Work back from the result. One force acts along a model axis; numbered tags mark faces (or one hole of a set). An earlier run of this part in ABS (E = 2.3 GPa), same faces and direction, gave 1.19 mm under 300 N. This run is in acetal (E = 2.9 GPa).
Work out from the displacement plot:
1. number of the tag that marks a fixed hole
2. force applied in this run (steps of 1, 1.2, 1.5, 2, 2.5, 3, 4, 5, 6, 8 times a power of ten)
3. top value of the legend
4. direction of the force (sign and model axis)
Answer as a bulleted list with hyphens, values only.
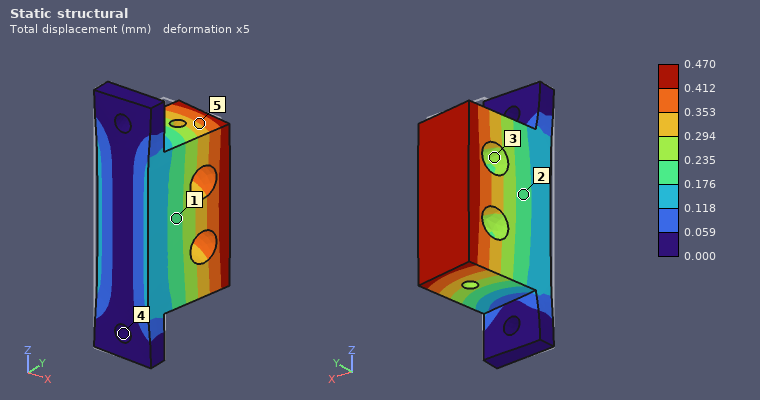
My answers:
- 4
- 150 N
- 0.470 mm
- +X
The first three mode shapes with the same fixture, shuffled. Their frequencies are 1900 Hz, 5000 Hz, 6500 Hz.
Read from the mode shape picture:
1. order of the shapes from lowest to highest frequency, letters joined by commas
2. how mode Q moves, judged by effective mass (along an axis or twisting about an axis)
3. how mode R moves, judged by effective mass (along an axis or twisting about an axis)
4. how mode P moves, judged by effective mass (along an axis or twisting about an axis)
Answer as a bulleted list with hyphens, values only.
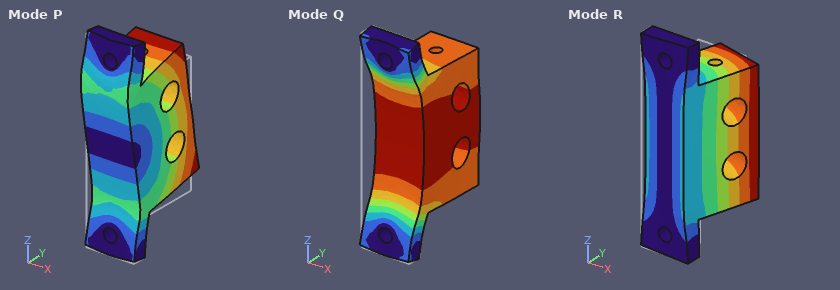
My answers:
- R, Q, P
- along Y
- along X
- along Z
